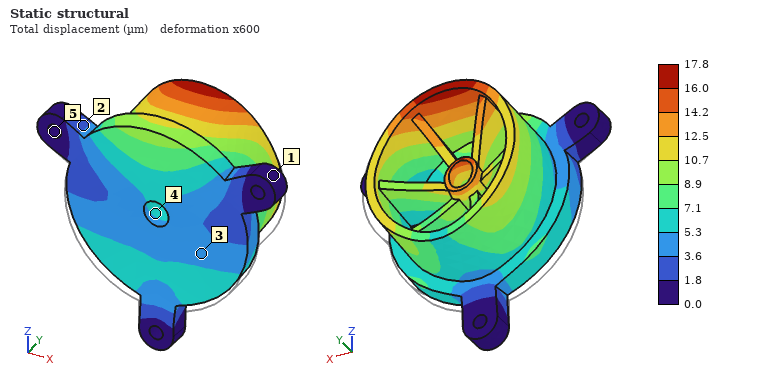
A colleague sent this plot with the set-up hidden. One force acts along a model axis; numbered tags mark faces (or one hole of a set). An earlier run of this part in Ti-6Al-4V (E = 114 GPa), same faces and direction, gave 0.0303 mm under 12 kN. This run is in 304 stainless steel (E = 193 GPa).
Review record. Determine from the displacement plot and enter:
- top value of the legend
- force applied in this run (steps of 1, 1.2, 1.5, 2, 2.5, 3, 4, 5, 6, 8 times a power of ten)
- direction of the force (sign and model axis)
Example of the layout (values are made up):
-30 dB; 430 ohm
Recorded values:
17.8 µm; 12 kN; +Z
